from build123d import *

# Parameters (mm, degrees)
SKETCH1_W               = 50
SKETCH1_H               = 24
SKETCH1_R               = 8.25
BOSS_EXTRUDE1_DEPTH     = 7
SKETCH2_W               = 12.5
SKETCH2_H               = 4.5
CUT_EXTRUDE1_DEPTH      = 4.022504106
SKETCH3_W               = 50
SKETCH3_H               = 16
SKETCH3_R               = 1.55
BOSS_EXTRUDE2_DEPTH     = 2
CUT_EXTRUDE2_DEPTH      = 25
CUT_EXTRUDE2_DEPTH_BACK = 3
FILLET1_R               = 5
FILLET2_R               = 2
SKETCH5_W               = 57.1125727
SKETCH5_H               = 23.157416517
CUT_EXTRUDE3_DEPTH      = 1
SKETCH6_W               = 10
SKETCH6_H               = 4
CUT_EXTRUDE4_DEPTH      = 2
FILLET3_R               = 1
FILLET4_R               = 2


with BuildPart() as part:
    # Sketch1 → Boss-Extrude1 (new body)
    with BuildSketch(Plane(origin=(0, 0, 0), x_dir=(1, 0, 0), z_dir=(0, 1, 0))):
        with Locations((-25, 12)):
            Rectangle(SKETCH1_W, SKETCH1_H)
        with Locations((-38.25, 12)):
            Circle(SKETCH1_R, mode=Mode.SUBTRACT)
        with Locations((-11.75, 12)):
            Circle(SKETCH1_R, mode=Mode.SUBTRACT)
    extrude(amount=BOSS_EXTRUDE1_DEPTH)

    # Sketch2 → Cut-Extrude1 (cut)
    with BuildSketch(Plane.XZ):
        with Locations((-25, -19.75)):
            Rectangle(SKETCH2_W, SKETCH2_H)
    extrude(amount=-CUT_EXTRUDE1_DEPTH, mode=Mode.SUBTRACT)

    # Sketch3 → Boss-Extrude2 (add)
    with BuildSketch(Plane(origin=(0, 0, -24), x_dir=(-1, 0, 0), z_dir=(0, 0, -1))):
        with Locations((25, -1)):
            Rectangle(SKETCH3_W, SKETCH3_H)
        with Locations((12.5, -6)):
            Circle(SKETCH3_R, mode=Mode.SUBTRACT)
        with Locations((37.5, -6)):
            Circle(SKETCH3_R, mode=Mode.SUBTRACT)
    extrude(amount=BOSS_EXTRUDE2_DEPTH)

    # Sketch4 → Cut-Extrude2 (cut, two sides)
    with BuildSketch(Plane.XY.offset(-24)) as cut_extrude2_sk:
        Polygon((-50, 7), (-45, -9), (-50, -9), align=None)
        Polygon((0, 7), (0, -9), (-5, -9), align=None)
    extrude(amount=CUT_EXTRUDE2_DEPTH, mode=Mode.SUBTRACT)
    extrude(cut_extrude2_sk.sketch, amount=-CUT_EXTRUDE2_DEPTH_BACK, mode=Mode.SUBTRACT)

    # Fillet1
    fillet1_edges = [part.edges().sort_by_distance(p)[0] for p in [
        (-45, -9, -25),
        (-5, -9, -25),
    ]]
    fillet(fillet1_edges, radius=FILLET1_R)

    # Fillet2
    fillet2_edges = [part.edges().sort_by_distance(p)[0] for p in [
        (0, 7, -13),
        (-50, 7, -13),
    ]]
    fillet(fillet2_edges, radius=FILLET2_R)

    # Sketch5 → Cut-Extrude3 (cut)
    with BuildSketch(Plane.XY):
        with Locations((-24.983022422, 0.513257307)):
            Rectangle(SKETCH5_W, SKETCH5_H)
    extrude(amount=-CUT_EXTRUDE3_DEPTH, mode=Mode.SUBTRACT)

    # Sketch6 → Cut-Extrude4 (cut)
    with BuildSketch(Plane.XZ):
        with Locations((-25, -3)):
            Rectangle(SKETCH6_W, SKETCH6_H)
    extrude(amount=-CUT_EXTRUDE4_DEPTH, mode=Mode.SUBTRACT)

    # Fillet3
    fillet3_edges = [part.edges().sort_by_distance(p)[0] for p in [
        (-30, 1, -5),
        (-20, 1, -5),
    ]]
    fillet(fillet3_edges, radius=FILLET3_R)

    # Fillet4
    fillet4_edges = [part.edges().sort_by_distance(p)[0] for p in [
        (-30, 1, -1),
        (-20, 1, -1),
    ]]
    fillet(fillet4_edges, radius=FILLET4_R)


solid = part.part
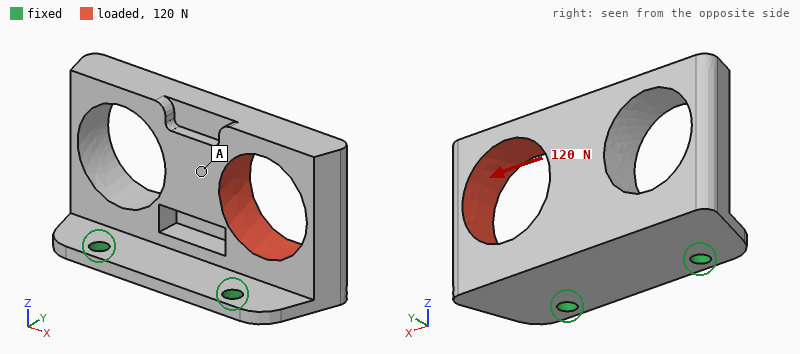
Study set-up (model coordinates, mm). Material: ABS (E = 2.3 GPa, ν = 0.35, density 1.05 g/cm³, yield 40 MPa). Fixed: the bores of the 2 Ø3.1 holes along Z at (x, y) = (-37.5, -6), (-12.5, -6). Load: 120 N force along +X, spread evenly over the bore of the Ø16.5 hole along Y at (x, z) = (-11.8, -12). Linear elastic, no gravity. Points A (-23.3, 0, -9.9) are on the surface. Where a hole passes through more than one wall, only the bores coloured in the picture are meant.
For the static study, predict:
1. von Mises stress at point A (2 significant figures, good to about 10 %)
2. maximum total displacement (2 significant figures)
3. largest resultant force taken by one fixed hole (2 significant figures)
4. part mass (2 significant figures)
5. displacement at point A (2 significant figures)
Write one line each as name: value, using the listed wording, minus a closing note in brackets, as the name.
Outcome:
von Mises stress at point A: 3.0 MPa
maximum total displacement: 0.46 mm
largest resultant force taken by one fixed hole: 93 N
part mass: 6.0 g
displacement at point A: 0.23 mm
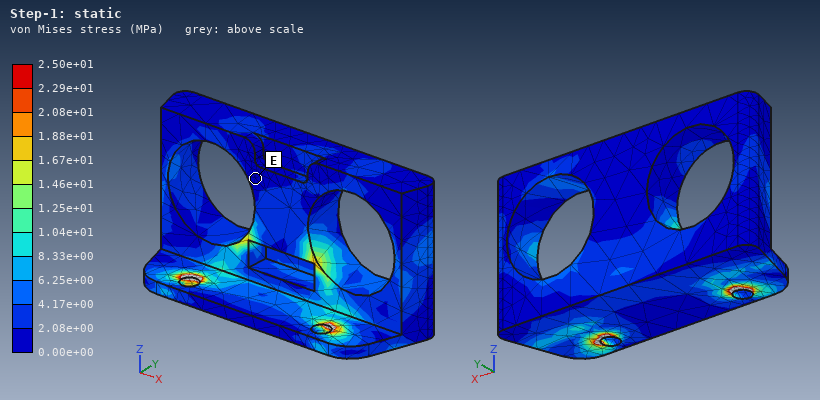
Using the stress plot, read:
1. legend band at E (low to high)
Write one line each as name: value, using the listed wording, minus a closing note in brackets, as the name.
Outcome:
legend band at E: 0.00e+00 to 2.08e+00 MPa
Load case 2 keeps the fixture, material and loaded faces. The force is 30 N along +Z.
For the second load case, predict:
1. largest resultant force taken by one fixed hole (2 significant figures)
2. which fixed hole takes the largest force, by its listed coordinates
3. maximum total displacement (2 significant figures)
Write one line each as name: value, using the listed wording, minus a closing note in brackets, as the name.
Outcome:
largest resultant force taken by one fixed hole: 29 N
which fixed hole takes the largest force, by its listed coordinates: (-12.5, -6)
maximum total displacement: 0.63 mm
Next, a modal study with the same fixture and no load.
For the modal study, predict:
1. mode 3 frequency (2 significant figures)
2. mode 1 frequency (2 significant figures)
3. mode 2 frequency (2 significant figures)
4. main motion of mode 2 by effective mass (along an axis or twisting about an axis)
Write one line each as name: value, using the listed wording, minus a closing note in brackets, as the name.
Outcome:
mode 3 frequency: 2200 Hz
mode 1 frequency: 420 Hz
mode 2 frequency: 1200 Hz
main motion of mode 2 by effective mass: along X
